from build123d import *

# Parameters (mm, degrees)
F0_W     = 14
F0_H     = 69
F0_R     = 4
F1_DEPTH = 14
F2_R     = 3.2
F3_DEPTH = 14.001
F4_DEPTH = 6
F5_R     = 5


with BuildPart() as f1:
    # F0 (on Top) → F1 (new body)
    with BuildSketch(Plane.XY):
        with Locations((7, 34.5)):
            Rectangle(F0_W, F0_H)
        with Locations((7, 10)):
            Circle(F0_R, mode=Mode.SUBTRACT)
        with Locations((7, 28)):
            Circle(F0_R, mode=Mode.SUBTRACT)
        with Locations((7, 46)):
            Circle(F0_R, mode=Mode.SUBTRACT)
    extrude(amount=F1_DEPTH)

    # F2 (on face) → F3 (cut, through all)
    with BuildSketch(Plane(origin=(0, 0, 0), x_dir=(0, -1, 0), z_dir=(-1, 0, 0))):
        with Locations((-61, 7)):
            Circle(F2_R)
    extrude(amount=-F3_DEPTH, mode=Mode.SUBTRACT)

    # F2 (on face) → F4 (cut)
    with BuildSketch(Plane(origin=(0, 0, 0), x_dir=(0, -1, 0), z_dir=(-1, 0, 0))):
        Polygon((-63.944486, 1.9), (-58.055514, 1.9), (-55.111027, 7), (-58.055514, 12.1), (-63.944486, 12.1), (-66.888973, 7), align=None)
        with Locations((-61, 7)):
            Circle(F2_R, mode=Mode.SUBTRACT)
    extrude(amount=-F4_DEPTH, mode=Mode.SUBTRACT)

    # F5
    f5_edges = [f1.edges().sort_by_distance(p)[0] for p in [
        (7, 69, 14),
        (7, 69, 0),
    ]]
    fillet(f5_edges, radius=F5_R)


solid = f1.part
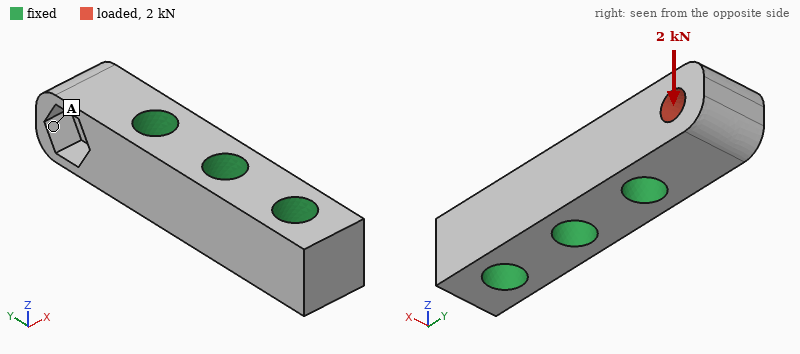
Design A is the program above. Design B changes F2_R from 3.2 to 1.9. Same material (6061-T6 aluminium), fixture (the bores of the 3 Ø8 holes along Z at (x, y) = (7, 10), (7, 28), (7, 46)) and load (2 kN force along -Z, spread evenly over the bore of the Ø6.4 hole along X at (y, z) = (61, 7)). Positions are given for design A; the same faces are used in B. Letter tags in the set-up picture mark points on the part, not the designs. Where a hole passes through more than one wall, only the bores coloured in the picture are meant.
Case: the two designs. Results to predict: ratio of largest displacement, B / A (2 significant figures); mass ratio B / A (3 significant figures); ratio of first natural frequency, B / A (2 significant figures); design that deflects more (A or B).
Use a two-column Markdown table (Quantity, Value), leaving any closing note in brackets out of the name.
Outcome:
| Quantity | Value |
|---|---|
| ratio of largest displacement, B / A | 0.81 |
| mass ratio B / A | 1.02 |
| ratio of first natural frequency, B / A | 1.0 |
| design that deflects more | A |
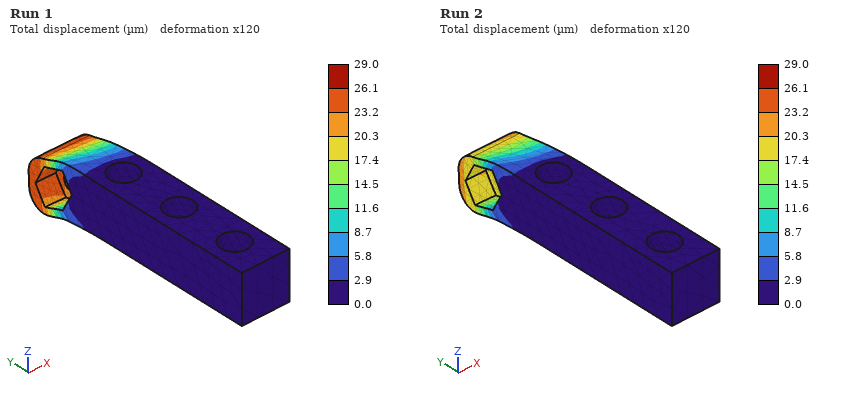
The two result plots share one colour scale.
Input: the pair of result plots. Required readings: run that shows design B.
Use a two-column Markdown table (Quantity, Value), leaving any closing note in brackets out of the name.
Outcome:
| Quantity | Value |
|---|---|
| run that shows design B | Run 2 |
